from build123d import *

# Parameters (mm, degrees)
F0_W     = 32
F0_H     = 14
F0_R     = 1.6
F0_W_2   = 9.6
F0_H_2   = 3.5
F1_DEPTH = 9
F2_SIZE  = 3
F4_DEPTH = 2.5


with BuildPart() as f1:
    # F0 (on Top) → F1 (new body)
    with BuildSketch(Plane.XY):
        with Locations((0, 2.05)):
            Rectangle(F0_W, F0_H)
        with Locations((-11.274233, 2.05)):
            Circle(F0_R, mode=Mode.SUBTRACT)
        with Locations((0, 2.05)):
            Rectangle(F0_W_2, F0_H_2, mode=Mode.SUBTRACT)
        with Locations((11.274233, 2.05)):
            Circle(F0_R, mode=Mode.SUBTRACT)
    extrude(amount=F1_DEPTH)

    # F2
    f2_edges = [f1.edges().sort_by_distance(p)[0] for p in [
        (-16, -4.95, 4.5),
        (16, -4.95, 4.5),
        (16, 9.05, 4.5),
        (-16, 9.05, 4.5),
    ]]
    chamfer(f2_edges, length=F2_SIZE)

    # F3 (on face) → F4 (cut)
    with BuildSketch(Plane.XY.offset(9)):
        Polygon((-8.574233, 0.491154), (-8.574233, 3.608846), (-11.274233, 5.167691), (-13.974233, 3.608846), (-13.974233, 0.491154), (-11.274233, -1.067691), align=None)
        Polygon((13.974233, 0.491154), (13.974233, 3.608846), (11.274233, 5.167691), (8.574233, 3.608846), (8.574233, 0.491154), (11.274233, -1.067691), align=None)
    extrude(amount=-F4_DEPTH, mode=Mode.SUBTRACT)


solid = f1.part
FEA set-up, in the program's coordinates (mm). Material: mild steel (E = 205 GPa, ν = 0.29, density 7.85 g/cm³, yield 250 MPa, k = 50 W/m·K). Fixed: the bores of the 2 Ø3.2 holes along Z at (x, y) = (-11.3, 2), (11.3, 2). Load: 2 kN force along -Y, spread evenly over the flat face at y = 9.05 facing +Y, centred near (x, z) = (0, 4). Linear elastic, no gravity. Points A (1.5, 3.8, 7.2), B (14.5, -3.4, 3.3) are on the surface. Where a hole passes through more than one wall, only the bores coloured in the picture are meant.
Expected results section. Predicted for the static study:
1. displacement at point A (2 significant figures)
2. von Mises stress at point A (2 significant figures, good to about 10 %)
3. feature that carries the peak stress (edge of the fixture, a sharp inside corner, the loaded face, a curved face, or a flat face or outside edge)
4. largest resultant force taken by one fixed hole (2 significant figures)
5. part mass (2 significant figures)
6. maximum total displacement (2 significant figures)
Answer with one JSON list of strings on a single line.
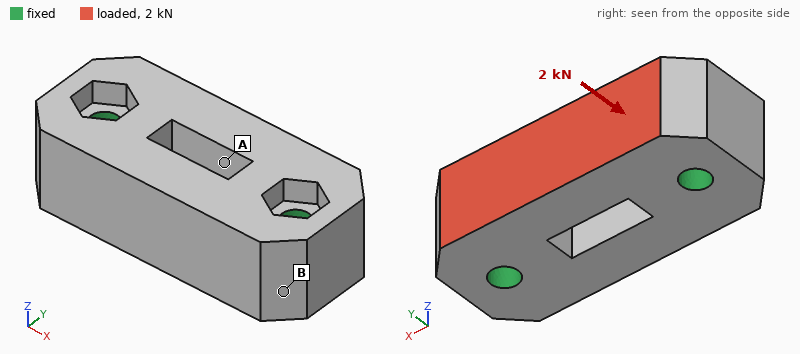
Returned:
["1.8 µm", "12 MPa", "edge of the fixture", "1.0 kN", "26 g", "2.2 µm"]
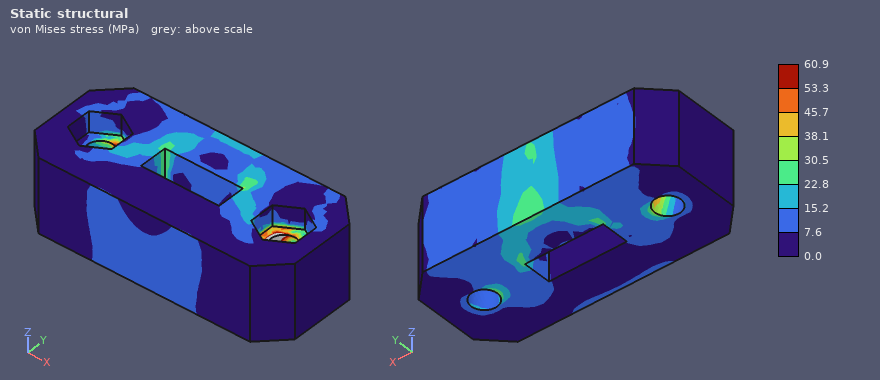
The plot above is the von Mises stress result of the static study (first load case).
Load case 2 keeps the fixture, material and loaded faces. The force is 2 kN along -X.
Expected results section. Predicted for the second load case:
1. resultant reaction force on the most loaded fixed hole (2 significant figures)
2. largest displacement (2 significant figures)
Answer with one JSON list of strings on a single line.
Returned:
["1.1 kN", "1.5 µm"]
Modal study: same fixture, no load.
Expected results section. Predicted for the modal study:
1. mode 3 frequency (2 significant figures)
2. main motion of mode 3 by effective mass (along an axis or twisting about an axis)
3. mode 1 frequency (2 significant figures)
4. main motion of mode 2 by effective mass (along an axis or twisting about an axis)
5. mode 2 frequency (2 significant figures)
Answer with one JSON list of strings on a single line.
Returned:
["52 kHz", "along Y", "40 kHz", "along Z", "44 kHz"]
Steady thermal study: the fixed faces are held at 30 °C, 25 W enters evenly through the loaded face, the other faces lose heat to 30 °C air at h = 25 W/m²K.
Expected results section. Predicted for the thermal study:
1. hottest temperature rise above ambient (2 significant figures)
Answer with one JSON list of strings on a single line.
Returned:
["29 K"]
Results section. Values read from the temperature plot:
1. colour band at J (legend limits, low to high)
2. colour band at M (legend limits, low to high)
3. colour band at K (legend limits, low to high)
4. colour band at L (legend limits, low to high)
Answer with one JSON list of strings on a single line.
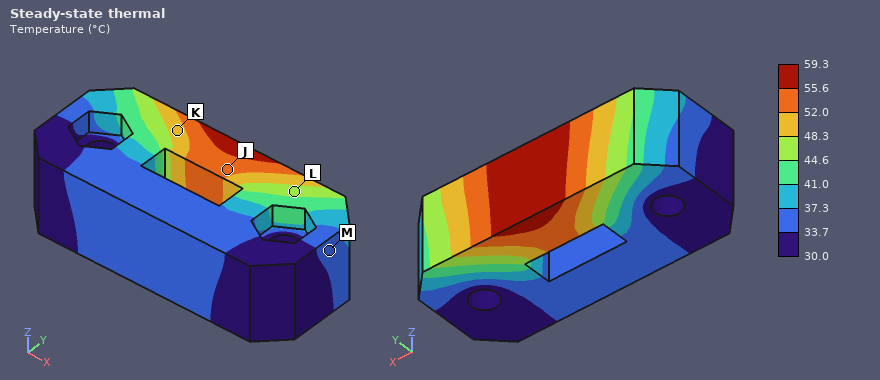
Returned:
["52.0 to 55.6 °C", "33.7 to 37.3 °C", "48.3 to 52.0 °C", "44.6 to 48.3 °C"]
